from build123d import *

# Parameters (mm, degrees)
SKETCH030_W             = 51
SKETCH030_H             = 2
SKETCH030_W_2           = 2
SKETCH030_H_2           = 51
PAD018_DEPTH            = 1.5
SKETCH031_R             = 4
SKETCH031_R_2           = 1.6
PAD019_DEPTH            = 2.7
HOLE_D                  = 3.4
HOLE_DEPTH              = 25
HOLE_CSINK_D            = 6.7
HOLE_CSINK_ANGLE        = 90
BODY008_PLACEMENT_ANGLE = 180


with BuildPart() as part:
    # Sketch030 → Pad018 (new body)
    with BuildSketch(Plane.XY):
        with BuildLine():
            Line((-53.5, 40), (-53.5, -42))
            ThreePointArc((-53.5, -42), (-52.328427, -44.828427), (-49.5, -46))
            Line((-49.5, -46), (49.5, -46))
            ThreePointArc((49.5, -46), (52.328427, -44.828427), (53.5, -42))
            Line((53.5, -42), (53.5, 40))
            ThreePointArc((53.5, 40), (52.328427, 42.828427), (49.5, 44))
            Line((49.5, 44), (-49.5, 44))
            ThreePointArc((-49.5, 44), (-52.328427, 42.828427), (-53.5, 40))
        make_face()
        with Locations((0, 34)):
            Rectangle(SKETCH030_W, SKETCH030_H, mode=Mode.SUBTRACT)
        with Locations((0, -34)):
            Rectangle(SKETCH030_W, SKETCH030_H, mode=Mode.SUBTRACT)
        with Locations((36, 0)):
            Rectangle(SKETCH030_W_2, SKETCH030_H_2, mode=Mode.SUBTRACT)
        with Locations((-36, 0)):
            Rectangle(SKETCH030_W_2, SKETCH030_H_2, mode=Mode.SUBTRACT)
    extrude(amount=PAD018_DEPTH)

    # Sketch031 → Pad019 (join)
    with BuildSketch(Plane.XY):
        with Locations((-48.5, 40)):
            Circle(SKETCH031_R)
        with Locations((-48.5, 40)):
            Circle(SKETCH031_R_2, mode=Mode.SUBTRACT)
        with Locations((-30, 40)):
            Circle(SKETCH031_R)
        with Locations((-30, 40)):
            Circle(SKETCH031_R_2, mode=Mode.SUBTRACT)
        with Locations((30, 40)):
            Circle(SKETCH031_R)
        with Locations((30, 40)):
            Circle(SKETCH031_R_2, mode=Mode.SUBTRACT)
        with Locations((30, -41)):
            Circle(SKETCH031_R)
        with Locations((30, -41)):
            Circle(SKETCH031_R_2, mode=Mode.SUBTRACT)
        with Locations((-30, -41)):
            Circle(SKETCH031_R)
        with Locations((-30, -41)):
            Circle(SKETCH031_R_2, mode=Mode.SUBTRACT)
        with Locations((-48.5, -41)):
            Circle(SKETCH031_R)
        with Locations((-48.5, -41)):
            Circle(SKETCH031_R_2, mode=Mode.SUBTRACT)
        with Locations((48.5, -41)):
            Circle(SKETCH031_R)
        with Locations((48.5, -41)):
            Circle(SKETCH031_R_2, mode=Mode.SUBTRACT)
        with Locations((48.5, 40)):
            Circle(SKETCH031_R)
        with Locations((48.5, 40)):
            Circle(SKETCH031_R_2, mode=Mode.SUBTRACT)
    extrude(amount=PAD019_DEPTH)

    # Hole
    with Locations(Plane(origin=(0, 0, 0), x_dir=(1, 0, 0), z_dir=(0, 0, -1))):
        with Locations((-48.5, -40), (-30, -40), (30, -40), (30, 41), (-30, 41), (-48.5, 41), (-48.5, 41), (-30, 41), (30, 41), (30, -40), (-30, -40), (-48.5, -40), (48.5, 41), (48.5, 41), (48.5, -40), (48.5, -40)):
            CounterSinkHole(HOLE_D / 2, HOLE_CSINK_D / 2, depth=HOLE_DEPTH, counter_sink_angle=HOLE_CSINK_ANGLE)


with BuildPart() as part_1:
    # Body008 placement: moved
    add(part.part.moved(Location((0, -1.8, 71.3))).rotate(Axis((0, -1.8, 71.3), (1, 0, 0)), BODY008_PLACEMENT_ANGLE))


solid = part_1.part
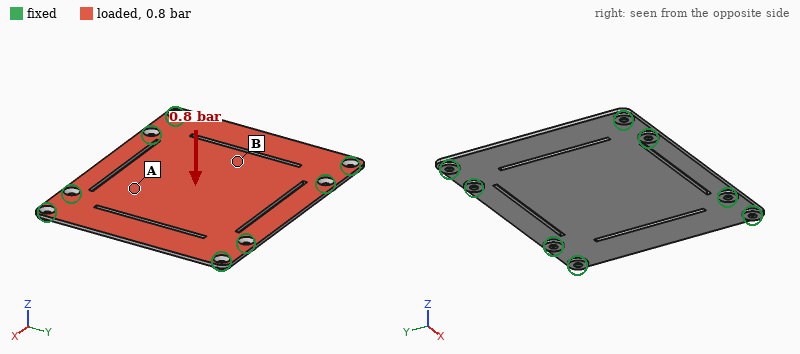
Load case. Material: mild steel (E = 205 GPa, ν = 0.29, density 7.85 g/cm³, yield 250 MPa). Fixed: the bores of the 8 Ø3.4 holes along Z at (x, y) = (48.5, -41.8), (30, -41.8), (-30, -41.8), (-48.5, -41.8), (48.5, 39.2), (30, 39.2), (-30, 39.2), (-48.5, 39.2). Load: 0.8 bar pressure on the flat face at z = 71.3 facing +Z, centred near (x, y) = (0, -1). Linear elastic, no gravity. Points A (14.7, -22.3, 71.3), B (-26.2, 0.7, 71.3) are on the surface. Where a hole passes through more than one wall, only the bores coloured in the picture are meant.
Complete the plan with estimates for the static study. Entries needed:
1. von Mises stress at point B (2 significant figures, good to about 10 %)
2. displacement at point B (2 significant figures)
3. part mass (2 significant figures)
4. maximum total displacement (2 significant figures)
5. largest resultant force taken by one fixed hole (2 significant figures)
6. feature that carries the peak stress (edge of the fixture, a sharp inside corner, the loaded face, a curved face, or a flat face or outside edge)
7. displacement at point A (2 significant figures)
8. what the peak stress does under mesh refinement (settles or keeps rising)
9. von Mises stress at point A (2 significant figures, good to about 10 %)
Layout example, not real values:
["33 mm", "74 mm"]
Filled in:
["76 MPa", "0.22 mm", "110 g", "0.27 mm", "300 N", "edge of the fixture", "0.17 mm", "keeps rising", "42 MPa"]
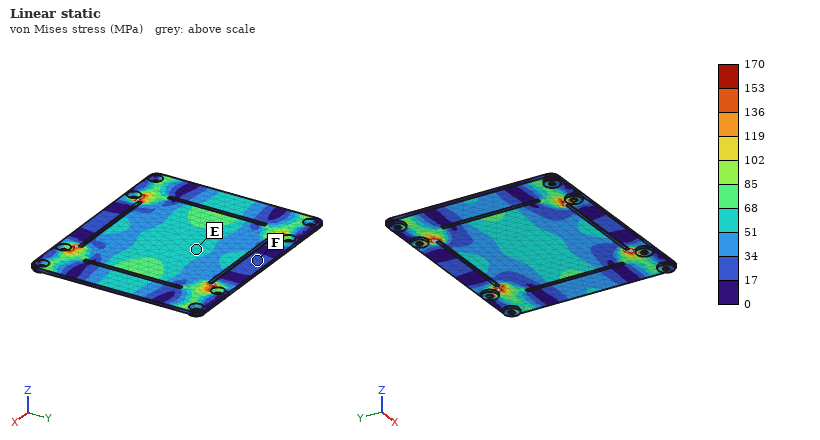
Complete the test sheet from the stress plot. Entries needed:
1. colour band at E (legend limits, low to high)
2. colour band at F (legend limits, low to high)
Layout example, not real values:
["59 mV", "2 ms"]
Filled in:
["51 to 68 MPa", "17 to 34 MPa"]
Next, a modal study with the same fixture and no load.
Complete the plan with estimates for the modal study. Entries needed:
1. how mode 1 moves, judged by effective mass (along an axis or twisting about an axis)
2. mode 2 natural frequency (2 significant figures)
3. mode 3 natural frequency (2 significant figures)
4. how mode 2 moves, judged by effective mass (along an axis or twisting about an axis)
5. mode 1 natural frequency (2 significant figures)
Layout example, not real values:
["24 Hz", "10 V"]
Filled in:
["along Z", "1400 Hz", "1500 Hz", "twisting about Y", "960 Hz"]
